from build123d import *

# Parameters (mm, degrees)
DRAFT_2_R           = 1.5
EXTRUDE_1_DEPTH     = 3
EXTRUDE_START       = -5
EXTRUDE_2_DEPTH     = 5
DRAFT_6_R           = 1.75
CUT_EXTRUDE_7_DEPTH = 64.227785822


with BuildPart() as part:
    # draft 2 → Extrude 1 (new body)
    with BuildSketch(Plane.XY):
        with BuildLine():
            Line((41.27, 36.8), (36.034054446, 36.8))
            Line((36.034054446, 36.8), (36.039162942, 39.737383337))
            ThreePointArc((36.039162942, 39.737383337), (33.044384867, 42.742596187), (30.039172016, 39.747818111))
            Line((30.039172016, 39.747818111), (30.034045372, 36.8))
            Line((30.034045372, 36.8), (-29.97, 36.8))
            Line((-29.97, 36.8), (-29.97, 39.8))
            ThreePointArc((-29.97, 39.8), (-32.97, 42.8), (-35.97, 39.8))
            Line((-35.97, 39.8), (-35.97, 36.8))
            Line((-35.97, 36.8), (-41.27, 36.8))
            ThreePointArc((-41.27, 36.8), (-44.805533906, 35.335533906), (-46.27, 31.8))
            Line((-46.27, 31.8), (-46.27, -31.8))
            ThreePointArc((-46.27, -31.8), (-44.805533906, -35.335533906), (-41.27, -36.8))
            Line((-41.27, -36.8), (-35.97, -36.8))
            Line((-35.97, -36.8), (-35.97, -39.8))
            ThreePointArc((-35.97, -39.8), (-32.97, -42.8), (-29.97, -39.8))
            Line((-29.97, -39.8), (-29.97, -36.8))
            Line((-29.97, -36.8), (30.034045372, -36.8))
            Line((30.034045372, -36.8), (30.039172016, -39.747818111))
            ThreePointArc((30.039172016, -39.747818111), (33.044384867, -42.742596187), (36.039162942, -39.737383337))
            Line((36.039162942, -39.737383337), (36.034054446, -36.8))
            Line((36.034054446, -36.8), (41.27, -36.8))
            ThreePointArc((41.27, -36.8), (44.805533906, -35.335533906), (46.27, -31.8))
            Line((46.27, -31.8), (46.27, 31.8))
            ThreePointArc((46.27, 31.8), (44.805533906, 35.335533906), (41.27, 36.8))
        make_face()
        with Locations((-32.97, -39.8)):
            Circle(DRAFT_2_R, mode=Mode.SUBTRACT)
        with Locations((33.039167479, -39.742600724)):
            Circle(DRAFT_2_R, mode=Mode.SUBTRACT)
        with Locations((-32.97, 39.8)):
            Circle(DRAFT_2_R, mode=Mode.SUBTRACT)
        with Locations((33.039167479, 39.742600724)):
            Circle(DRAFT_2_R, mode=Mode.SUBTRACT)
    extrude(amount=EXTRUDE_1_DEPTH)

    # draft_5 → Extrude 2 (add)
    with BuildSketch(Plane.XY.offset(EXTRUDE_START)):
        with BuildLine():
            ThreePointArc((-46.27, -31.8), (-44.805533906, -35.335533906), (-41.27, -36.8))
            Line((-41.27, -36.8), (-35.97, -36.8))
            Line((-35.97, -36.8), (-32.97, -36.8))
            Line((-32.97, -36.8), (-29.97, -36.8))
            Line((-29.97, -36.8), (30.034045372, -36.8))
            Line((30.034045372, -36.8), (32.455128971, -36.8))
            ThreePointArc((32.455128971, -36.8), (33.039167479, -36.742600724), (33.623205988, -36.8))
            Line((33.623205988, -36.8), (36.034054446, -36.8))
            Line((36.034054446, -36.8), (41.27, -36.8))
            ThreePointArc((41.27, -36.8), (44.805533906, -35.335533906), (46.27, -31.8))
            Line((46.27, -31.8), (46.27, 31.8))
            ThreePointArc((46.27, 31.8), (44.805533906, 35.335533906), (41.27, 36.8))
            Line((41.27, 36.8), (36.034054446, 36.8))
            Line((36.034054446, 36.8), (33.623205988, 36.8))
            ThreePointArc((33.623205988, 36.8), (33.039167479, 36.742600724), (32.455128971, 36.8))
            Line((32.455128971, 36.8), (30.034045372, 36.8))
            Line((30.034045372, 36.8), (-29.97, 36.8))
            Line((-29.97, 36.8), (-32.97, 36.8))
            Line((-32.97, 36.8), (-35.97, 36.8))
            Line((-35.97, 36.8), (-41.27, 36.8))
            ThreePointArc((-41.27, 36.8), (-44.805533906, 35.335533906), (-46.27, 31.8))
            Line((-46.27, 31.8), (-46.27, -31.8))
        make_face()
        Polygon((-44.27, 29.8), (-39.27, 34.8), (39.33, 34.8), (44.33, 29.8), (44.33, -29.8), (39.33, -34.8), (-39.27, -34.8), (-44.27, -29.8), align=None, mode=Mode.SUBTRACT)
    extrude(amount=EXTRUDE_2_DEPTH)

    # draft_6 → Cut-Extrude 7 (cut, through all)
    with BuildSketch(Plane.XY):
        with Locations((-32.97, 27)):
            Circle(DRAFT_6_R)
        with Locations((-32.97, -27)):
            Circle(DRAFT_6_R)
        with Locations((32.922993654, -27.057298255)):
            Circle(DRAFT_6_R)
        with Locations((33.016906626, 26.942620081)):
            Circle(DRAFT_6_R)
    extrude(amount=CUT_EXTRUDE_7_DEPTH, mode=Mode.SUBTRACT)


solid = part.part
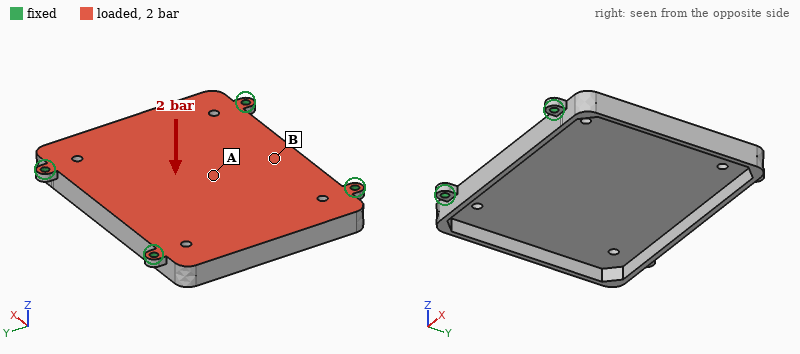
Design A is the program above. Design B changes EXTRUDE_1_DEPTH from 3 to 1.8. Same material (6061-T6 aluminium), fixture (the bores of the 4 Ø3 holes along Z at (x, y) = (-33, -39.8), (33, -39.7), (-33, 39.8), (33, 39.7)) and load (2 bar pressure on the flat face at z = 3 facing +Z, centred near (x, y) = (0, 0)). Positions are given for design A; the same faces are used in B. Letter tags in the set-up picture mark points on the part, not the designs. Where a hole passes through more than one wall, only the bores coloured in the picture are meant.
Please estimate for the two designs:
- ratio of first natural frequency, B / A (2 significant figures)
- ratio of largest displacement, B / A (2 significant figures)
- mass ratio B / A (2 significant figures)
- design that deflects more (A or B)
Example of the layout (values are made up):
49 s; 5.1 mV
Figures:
0.71; 3.4; 0.66; B
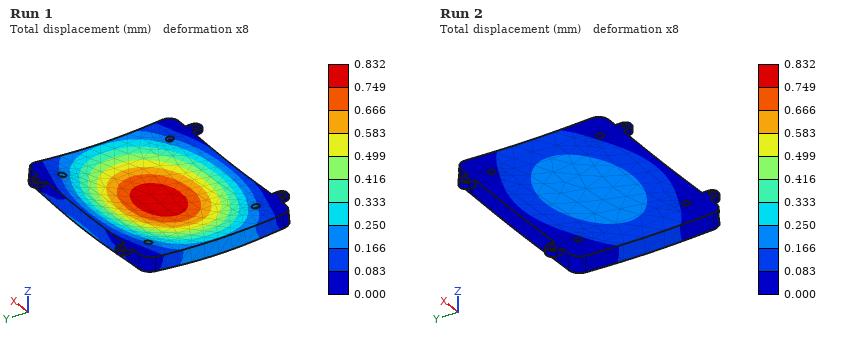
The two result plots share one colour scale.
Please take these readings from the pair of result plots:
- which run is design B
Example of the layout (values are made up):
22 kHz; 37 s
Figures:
Run 1
